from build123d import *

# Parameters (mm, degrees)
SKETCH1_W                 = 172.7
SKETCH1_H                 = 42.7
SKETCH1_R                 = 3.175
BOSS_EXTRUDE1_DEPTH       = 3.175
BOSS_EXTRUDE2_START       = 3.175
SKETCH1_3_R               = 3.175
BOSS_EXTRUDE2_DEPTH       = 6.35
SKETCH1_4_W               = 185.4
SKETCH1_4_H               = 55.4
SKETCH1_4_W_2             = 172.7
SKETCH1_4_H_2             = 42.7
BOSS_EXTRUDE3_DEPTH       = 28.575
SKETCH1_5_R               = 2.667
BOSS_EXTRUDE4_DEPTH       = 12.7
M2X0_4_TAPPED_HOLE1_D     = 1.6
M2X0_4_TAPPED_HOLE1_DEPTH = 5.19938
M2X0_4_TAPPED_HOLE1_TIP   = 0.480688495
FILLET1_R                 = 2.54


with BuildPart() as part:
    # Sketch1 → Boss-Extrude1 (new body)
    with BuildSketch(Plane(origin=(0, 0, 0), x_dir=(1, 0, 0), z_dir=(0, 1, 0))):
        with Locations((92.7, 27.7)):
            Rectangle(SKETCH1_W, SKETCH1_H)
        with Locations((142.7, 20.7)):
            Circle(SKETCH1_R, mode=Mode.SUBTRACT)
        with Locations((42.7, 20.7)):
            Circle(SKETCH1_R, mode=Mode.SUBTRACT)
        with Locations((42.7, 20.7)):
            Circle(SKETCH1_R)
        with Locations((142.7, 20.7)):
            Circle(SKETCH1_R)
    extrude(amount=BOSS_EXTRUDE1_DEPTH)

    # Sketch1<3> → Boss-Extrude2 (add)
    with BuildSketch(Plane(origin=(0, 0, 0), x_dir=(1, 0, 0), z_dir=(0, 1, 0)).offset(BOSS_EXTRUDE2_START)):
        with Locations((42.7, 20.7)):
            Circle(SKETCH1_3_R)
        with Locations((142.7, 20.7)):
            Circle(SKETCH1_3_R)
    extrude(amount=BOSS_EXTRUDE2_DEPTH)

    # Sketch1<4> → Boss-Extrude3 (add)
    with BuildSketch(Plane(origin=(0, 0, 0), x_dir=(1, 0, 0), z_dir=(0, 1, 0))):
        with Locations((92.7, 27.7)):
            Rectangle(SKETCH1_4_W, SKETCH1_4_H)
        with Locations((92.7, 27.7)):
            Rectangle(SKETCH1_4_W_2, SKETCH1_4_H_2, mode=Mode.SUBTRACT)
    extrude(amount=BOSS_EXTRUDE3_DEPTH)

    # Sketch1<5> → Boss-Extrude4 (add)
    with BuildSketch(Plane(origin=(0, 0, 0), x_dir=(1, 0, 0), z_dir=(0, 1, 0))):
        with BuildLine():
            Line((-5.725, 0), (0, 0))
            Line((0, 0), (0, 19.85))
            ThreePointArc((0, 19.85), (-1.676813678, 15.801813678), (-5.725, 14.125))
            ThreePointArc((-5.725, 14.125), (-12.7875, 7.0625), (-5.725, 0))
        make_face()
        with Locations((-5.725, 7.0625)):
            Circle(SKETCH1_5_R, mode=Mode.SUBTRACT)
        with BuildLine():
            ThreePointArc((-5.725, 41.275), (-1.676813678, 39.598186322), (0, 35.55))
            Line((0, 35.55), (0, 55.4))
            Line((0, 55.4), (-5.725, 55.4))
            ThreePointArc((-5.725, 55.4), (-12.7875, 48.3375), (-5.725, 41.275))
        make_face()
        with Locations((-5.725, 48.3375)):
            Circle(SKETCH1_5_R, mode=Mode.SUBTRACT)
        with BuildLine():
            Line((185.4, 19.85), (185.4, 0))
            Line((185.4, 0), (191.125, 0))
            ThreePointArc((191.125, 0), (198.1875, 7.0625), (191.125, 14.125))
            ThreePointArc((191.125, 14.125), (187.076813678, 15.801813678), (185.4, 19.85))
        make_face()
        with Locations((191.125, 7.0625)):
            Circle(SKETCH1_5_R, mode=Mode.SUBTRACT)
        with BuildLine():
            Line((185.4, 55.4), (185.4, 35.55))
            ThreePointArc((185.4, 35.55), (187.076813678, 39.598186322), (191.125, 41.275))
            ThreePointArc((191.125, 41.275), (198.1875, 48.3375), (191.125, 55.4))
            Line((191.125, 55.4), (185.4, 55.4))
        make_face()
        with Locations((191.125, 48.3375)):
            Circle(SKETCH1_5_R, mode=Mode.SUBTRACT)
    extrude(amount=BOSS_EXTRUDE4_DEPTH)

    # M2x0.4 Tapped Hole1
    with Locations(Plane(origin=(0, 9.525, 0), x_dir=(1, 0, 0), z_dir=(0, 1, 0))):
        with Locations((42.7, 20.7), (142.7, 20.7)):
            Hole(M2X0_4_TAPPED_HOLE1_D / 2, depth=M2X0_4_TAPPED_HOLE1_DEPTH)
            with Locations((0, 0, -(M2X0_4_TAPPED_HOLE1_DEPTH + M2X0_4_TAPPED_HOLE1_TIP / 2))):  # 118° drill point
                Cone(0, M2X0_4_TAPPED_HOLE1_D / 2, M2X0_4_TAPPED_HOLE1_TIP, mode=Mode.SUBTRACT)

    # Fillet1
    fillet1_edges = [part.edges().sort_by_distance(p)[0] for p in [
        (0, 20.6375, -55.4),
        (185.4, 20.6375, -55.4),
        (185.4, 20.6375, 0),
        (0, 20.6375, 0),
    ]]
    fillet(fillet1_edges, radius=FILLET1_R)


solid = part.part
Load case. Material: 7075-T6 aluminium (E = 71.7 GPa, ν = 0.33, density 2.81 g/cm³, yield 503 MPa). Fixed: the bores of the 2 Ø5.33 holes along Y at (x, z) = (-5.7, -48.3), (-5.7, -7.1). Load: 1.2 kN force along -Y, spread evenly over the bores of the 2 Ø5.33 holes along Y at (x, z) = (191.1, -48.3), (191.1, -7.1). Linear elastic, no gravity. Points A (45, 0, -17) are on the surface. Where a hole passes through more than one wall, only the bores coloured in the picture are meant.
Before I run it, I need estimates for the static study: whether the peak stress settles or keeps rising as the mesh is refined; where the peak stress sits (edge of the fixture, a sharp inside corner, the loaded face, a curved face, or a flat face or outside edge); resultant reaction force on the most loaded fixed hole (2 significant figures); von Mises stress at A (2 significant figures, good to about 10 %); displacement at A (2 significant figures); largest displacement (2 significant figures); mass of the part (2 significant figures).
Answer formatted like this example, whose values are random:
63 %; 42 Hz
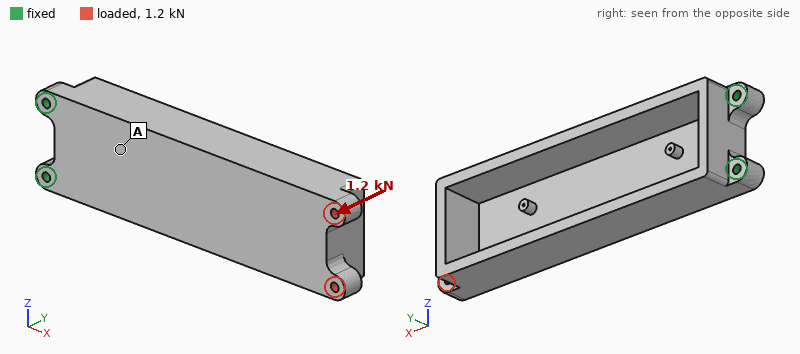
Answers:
keeps rising; edge of the fixture; 2.0 kN; 46 MPa; 0.43 mm; 2.5 mm; 320 g
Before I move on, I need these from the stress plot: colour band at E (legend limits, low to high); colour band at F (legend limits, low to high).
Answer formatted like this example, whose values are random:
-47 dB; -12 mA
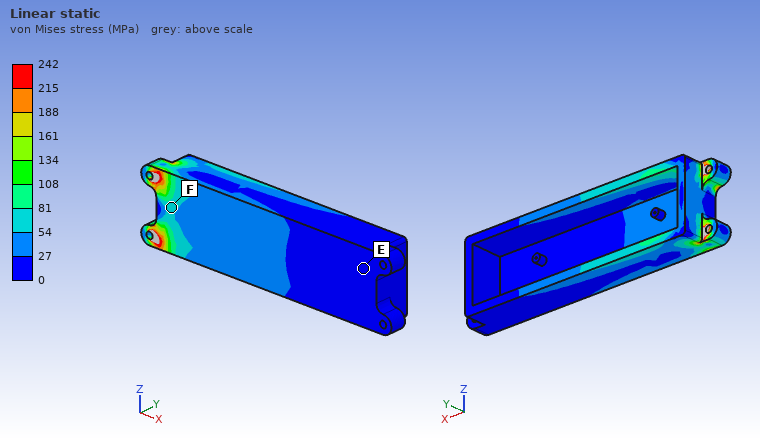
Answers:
0 to 27 MPa; 54 to 81 MPa
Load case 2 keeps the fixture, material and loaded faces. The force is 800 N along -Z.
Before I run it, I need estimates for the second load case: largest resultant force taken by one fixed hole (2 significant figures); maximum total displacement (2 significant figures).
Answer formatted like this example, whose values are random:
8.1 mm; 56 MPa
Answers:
3.6 kN; 0.43 mm
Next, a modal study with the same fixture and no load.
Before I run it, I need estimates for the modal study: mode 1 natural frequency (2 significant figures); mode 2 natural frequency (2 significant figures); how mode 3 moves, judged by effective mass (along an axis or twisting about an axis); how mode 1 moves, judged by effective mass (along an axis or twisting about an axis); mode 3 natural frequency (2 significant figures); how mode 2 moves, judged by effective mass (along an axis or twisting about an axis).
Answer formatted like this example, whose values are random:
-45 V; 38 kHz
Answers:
350 Hz; 590 Hz; along Z; along Y; 1300 Hz; along Z
